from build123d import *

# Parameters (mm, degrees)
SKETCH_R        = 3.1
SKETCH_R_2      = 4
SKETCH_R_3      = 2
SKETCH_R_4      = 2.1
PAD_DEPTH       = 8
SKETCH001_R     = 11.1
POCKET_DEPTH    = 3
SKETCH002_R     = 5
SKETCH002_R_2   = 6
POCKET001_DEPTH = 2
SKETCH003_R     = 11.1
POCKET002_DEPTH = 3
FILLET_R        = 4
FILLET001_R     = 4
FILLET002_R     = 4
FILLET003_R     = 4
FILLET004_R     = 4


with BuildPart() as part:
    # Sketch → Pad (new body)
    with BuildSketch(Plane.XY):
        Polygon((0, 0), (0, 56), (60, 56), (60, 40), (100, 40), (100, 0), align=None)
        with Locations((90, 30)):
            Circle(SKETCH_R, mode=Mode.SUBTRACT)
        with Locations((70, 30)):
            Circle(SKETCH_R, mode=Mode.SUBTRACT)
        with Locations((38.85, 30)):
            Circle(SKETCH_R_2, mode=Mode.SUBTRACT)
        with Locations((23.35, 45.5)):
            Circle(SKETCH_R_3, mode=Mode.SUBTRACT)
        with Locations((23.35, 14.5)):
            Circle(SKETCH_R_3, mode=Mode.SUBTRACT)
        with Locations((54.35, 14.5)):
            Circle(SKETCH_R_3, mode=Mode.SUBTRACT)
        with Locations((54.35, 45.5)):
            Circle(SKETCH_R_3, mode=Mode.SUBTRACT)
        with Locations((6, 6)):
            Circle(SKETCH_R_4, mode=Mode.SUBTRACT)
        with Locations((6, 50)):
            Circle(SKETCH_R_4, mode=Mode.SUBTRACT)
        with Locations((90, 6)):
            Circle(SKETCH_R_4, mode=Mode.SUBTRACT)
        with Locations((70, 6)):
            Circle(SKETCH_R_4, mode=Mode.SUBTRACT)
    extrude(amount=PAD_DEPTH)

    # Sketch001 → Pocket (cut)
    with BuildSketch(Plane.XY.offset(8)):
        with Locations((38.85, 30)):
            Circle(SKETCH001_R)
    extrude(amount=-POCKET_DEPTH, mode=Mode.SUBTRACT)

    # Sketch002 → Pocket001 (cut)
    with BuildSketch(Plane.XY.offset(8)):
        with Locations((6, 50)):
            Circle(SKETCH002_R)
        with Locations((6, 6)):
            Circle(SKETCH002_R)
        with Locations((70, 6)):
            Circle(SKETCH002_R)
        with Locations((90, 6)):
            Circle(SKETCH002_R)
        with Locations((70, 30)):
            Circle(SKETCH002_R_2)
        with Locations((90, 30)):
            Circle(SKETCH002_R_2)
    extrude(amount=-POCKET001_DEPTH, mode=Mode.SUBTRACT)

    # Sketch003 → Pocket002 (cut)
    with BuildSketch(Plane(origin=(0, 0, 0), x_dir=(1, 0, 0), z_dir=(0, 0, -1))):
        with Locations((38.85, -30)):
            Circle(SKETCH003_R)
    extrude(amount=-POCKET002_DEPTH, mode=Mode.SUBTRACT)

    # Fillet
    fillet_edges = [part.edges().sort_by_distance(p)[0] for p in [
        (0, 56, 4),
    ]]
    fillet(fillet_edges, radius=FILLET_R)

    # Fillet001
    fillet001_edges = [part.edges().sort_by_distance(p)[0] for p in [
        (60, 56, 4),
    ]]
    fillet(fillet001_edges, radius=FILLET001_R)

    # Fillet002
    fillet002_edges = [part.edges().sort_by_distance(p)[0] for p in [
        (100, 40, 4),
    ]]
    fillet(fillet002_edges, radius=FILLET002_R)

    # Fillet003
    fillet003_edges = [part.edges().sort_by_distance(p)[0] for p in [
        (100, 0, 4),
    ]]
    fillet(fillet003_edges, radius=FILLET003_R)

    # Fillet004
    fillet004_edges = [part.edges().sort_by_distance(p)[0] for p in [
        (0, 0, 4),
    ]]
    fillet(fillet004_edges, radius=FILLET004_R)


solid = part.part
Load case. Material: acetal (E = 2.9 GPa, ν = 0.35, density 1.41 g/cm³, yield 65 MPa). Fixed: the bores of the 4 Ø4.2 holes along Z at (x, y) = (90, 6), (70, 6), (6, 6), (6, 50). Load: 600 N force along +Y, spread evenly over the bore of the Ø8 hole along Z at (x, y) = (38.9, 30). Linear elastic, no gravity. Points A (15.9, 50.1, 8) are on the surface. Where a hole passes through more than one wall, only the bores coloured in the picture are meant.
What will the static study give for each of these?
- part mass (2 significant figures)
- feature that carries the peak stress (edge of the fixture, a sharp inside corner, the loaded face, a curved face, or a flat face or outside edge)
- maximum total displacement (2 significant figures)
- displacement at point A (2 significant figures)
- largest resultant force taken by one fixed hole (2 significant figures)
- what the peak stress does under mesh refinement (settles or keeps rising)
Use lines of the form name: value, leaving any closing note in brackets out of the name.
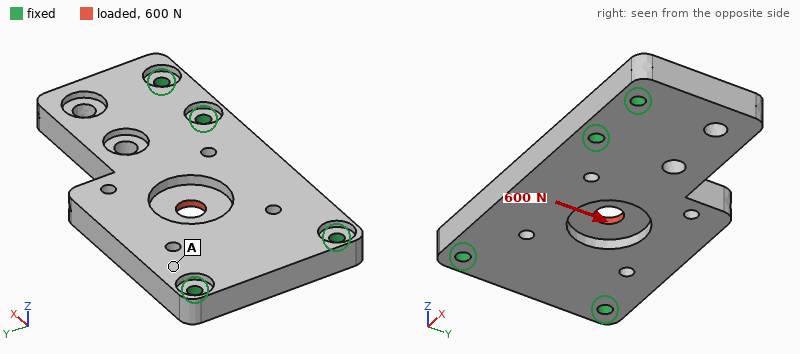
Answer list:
part mass: 49 g
feature that carries the peak stress: a sharp inside corner
maximum total displacement: 67 µm
displacement at point A: 13 µm
largest resultant force taken by one fixed hole: 260 N
what the peak stress does under mesh refinement: keeps rising
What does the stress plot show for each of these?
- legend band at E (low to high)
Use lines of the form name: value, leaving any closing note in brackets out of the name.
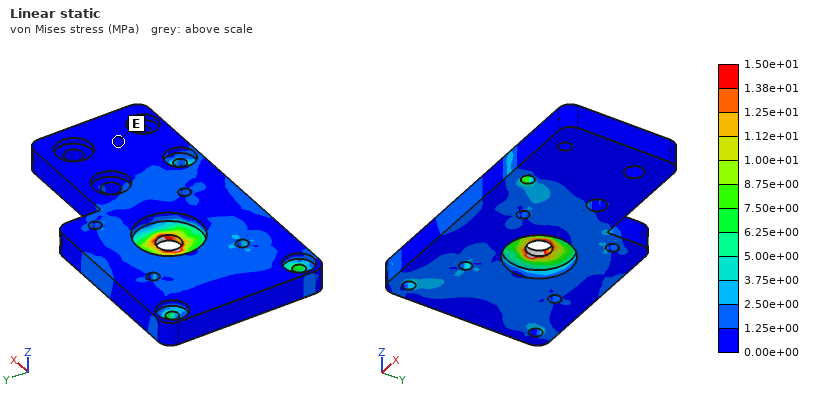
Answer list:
legend band at E: 0.00e+00 to 1.25e+00 MPa
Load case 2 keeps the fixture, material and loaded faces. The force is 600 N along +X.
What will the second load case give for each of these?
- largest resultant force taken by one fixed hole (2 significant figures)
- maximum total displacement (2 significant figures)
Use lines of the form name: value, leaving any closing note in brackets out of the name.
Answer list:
largest resultant force taken by one fixed hole: 200 N
maximum total displacement: 53 µm
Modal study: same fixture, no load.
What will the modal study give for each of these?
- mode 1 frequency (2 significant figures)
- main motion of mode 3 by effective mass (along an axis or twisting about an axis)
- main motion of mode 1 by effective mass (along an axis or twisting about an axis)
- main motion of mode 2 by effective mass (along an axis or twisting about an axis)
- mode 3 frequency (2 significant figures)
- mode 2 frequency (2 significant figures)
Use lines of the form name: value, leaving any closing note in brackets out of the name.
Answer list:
mode 1 frequency: 1100 Hz
main motion of mode 3 by effective mass: along Z
main motion of mode 1 by effective mass: along Z
main motion of mode 2 by effective mass: twisting about Y
mode 3 frequency: 2400 Hz
mode 2 frequency: 1800 Hz
